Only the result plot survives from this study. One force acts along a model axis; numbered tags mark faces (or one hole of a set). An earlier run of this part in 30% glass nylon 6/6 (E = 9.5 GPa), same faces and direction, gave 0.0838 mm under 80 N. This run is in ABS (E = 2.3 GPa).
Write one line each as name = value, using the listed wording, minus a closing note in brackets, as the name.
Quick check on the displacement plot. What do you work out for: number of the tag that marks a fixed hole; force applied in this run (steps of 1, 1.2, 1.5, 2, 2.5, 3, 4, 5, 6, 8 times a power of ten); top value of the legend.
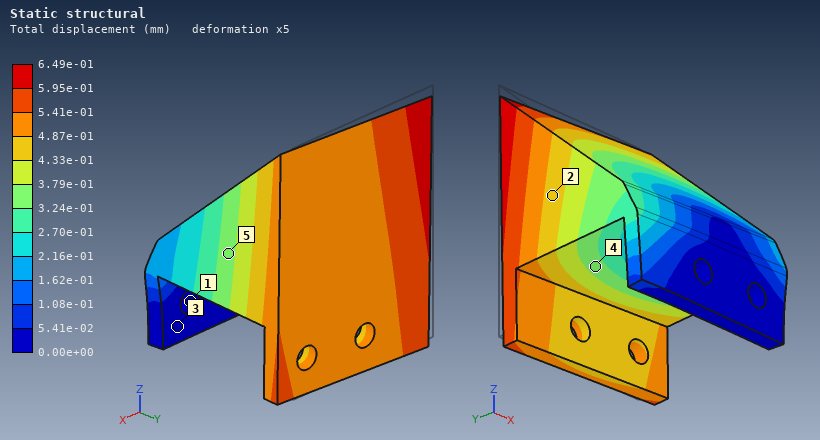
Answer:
number of the tag that marks a fixed hole = 1
force applied in this run = 150 N
top value of the legend = 6.49e-01 mm
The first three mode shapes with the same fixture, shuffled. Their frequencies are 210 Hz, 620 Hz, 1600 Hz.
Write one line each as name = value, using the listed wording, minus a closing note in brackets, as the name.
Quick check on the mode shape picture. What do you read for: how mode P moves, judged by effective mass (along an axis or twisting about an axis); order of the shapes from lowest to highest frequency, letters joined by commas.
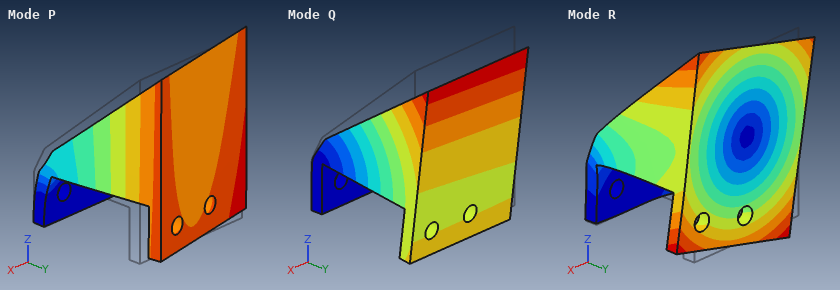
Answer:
how mode P moves, judged by effective mass = along X
order of the shapes from lowest to highest frequency, letters joined by commas = Q, P, R
